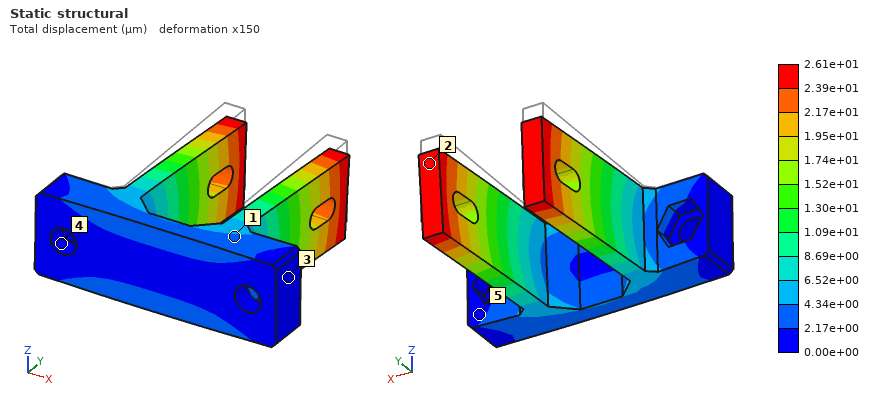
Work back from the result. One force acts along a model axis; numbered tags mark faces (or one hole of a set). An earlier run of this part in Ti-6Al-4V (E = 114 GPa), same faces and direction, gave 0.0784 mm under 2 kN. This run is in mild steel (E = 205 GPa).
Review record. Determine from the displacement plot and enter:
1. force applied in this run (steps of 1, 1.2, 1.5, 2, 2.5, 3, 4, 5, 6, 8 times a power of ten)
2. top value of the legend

1.2 kN
2.61e+01 µm
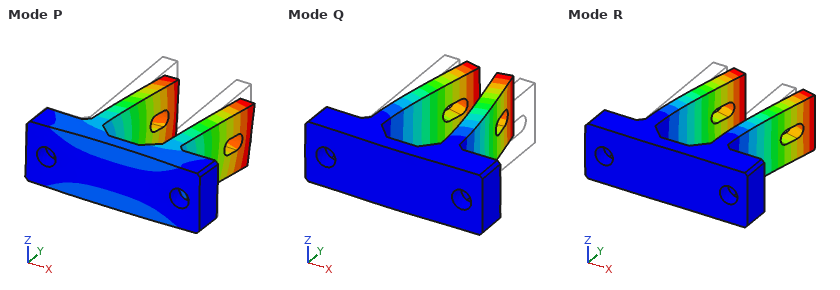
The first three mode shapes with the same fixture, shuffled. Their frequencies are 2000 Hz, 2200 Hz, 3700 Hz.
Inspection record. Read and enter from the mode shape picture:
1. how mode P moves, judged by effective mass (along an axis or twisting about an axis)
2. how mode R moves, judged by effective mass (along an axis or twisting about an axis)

along Z
along X
